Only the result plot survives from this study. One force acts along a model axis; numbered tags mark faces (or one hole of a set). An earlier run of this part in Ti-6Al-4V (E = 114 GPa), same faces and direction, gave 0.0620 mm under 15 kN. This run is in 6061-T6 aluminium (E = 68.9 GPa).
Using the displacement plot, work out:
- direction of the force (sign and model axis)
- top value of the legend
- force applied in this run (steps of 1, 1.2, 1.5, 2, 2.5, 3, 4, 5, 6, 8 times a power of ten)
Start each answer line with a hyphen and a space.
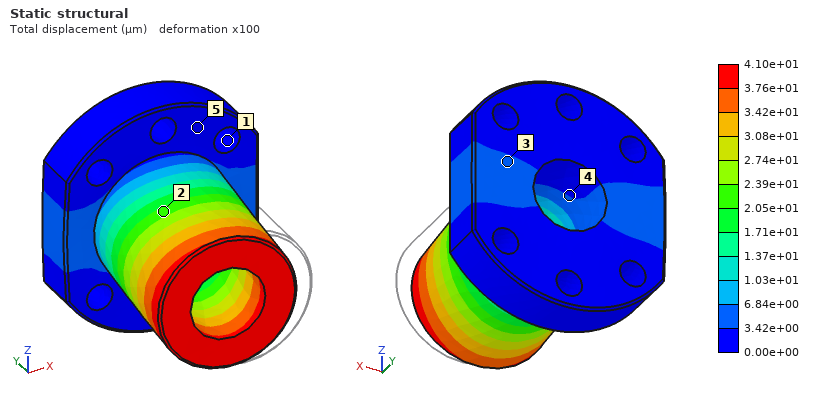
- -X
- 4.10e+01 µm
- 6 kN
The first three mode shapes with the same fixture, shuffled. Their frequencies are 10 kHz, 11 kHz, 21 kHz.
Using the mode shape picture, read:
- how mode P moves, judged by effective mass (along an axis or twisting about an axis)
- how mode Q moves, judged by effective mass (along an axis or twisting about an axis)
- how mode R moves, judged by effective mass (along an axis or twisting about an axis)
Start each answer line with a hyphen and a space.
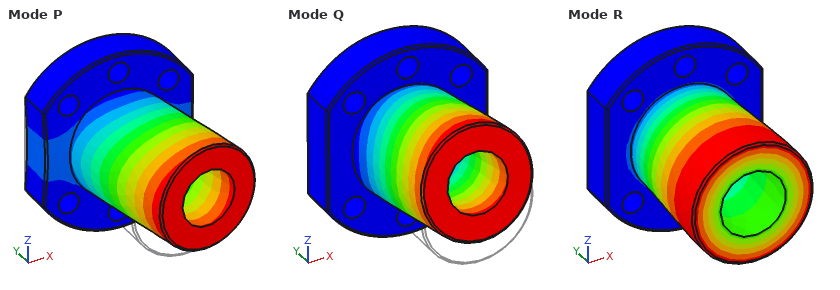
- along X
- along Z
- twisting about Y
